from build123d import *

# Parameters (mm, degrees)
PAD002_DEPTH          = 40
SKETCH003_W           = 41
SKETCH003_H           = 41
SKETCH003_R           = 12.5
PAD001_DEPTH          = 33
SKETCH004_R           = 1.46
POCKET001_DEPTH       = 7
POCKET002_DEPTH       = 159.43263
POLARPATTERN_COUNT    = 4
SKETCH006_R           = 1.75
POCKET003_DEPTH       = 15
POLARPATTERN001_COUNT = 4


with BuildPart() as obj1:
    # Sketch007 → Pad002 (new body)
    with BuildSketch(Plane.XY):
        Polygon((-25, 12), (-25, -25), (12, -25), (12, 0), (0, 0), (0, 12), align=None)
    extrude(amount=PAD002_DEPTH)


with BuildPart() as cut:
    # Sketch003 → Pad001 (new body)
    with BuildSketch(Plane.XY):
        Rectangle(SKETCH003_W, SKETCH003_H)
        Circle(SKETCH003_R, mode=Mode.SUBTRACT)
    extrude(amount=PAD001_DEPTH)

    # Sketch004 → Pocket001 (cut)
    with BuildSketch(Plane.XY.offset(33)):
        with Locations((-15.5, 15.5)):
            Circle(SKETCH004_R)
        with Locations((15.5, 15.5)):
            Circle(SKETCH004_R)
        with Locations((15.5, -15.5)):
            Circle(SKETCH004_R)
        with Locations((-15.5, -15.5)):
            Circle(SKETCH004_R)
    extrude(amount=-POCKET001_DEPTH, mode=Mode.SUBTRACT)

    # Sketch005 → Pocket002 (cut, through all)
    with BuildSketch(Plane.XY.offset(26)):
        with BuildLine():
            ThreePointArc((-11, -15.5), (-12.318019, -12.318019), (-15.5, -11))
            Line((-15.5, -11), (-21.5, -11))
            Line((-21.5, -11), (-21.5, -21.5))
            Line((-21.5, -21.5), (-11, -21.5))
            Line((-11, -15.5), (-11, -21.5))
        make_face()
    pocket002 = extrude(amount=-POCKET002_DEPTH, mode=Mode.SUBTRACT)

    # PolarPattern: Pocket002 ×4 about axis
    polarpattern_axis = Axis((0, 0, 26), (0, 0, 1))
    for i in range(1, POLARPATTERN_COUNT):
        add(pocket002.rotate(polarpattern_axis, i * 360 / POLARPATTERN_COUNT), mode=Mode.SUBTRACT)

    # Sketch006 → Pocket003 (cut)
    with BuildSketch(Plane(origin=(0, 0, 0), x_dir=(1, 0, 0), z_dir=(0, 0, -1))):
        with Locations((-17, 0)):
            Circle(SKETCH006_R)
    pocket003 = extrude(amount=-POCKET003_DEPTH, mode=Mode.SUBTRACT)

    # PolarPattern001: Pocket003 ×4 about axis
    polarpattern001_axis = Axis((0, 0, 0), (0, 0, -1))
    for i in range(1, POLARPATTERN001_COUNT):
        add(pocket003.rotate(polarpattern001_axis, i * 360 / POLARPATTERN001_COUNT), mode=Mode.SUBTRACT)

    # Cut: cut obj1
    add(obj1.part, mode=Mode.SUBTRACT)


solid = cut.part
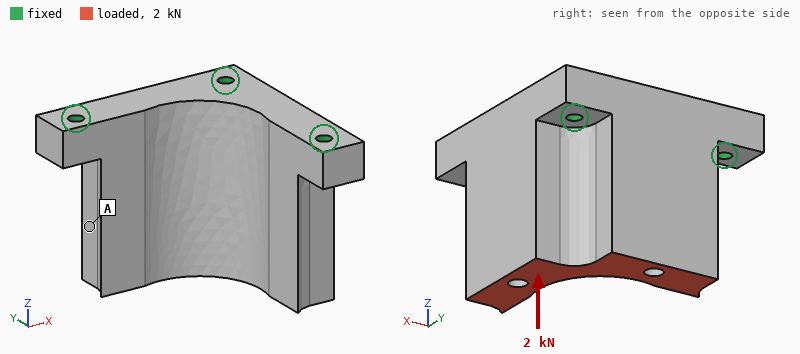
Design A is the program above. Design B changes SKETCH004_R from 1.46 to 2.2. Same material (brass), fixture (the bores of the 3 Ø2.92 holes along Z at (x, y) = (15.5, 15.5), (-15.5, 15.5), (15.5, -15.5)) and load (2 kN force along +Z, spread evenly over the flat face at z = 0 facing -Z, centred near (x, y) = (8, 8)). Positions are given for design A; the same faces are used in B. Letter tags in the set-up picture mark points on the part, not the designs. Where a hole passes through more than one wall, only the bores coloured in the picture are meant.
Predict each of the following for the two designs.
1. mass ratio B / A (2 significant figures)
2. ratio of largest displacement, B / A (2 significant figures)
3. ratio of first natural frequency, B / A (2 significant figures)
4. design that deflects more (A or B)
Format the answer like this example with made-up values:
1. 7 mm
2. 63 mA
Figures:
1. 0.99
2. 0.85
3. 1.1
4. A
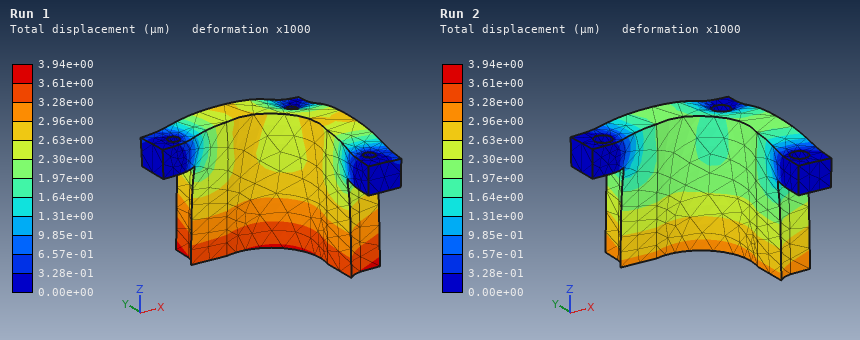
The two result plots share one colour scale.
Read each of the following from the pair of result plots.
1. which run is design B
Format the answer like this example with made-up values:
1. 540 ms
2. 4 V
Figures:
1. Run 2
